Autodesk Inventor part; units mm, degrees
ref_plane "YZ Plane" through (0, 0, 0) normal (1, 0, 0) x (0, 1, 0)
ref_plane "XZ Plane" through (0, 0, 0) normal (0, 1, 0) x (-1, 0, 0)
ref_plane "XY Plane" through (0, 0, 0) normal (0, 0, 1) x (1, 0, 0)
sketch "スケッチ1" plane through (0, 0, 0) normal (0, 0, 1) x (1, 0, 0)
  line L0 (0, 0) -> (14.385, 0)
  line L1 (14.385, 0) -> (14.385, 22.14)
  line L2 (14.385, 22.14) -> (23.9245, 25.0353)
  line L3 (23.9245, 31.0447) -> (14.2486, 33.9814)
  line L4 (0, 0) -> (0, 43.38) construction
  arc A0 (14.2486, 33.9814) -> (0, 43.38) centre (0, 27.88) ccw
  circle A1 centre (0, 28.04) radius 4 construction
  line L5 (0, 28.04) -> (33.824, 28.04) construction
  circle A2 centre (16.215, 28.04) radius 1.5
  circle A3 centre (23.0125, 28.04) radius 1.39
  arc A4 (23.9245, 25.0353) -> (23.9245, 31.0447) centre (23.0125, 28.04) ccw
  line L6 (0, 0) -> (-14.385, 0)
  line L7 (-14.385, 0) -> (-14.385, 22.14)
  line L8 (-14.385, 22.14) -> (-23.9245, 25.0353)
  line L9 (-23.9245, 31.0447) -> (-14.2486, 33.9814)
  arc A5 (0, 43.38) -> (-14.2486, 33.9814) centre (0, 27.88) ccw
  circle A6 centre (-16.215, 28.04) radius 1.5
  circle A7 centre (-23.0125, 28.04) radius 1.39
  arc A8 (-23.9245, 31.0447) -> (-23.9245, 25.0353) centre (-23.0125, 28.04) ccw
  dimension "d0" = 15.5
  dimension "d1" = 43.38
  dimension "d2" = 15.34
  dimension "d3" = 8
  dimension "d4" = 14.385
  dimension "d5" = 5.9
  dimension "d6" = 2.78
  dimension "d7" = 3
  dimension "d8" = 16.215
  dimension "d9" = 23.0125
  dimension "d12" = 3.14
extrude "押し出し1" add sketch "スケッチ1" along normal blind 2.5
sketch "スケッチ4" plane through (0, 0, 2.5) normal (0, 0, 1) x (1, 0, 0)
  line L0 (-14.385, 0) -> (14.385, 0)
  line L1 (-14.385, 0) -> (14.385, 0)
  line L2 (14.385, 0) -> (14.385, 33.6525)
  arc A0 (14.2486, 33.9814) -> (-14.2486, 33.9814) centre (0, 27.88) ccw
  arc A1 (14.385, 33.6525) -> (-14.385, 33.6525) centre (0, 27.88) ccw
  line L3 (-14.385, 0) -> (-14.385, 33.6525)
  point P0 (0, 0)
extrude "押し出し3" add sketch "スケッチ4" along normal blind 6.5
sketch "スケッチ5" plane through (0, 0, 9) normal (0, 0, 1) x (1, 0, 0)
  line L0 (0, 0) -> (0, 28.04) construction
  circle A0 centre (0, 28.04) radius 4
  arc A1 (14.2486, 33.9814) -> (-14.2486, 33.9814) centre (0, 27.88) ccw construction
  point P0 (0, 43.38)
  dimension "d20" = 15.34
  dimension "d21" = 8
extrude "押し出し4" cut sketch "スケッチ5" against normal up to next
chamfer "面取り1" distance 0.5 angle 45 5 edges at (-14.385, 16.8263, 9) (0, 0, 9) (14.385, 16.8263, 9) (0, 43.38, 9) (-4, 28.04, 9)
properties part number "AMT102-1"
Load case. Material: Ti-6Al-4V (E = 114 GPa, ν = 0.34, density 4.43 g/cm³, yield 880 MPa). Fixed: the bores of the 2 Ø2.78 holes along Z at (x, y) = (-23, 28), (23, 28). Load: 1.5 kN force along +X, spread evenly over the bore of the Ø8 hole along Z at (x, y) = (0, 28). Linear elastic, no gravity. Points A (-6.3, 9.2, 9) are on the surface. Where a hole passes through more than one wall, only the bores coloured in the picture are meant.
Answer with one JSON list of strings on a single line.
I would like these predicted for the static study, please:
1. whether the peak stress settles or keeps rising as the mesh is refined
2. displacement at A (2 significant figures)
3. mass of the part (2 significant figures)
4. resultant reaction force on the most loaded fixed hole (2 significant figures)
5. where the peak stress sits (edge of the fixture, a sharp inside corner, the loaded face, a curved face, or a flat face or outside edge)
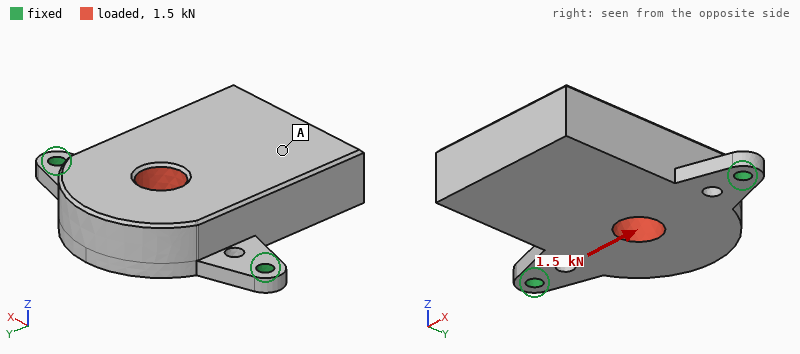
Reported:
["keeps rising", "6.9 µm", "46 g", "760 N", "edge of the fixture"]
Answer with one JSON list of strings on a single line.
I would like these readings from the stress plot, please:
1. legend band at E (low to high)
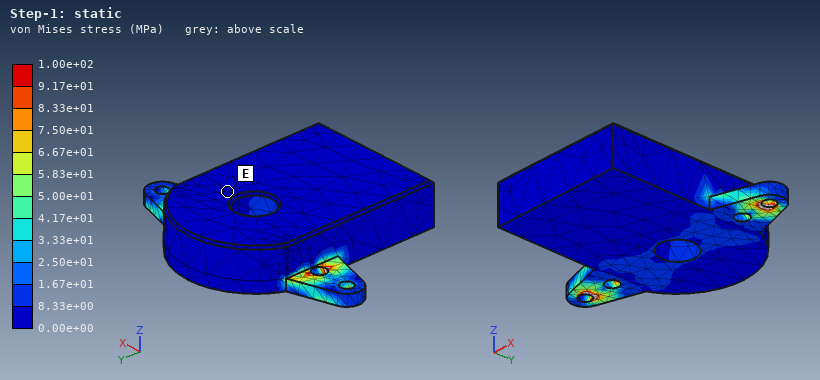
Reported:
["0.00e+00 to 8.33e+00 MPa"]
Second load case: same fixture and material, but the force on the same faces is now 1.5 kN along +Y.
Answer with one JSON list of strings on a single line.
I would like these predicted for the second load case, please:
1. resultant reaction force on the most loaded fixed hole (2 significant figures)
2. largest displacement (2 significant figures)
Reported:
["750 N", "0.30 mm"]
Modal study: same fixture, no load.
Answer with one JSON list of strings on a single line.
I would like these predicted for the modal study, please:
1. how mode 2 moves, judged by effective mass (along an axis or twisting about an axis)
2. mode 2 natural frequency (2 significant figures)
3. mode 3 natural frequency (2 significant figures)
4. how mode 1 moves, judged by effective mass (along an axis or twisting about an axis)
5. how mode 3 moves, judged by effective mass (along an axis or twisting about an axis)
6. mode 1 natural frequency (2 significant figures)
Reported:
["along Z", "4700 Hz", "7500 Hz", "along Z", "along X", "1100 Hz"]
